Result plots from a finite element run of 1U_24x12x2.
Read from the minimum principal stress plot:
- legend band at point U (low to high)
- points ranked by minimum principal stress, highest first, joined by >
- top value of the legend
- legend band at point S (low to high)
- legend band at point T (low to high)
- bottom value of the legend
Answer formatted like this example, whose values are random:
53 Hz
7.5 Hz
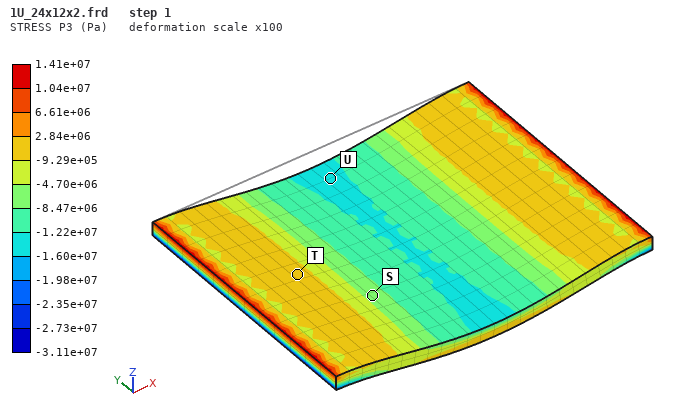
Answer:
-1.60e+07 to -1.22e+07 Pa
T > S > U
1.41e+07 Pa
-8.47e+06 to -4.70e+06 Pa
-9.29e+05 to 2.84e+06 Pa
-3.11e+07 Pa
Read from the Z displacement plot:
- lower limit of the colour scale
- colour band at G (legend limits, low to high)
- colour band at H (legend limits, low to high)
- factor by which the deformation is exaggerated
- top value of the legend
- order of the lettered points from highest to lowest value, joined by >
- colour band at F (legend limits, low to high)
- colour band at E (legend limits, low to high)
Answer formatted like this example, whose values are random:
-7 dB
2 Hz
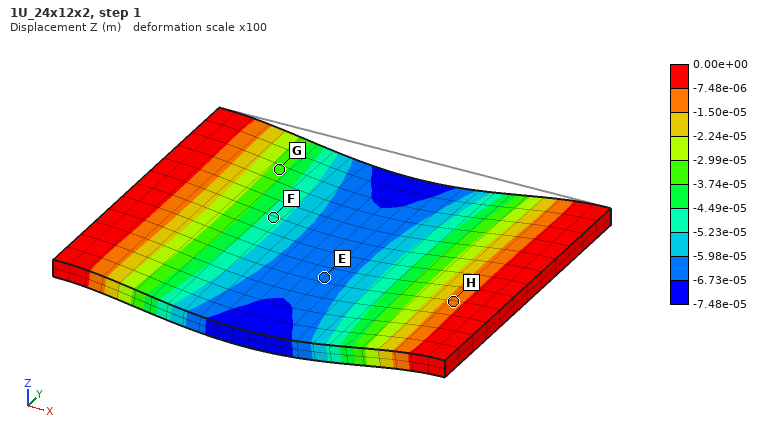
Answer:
-7.48e-05 m
-3.74e-05 to -2.99e-05 m
-1.50e-05 to -7.48e-06 m
100
0.00e+00 m
H > G > F > E
-5.23e-05 to -4.49e-05 m
-6.73e-05 to -5.98e-05 m
